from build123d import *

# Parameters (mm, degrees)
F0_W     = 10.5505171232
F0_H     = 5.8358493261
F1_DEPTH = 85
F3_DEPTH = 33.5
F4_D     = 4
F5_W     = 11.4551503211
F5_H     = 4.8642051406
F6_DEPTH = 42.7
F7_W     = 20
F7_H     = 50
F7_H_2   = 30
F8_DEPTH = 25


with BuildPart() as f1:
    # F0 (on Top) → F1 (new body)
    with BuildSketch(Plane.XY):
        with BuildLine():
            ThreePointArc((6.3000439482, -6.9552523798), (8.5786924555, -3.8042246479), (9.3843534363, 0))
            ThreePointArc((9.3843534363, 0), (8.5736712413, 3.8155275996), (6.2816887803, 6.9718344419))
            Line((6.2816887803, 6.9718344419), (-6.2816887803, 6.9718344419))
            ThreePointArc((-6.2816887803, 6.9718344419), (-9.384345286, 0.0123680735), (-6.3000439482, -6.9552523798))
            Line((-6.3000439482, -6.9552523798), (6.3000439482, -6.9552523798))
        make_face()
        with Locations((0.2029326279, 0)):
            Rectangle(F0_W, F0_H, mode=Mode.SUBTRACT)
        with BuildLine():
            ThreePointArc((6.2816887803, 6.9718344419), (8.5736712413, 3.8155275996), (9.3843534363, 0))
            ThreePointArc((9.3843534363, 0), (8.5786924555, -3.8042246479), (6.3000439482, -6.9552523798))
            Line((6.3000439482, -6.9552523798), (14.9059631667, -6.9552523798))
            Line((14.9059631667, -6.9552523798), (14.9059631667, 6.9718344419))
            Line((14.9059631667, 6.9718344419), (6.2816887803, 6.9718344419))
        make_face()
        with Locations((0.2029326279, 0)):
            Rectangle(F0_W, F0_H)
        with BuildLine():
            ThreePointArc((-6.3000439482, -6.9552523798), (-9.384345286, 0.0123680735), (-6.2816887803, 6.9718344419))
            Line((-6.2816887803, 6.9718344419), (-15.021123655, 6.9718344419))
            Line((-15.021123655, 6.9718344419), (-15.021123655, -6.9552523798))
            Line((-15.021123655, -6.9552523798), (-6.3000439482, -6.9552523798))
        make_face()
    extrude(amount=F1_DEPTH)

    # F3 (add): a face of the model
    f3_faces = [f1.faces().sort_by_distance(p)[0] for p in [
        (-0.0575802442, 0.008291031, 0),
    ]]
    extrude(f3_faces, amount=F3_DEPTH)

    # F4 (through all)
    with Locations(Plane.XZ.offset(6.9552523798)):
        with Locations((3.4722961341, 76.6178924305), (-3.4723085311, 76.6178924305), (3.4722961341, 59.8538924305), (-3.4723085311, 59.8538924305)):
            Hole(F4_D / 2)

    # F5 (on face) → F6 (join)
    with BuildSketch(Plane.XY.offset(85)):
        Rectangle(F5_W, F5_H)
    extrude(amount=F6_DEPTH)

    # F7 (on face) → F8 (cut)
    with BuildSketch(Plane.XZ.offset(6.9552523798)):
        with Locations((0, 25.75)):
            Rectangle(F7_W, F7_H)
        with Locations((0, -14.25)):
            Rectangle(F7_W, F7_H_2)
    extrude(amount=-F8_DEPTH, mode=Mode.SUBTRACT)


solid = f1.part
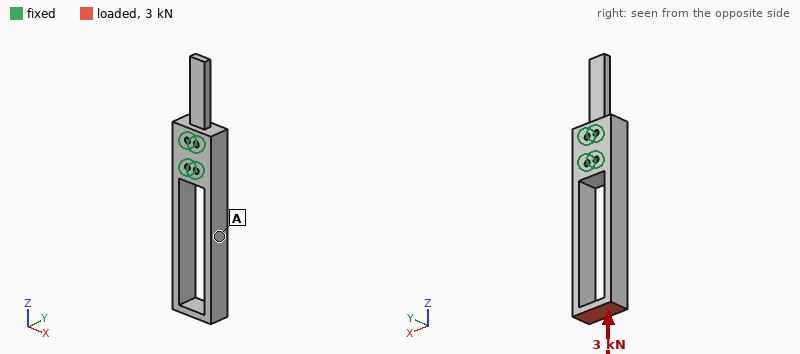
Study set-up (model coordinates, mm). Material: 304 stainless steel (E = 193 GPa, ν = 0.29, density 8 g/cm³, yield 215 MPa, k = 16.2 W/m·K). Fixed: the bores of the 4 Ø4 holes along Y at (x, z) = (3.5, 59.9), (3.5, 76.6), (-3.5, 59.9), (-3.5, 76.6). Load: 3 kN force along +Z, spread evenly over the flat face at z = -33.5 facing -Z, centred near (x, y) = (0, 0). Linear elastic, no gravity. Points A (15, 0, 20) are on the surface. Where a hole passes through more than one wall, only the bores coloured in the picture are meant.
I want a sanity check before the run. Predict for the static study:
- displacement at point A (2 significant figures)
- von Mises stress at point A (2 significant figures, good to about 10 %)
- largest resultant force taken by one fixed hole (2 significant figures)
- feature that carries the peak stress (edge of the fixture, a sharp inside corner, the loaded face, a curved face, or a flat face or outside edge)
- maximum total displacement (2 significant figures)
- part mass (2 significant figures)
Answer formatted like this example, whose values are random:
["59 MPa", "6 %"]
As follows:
["21 µm", "16 MPa", "920 N", "a flat face or outside edge", "30 µm", "230 g"]
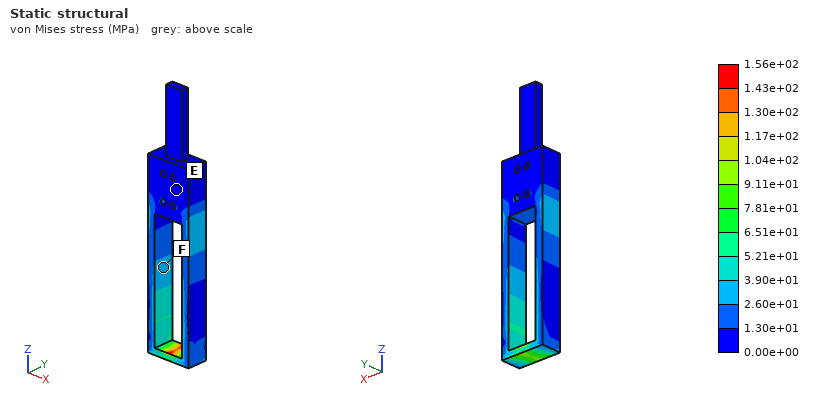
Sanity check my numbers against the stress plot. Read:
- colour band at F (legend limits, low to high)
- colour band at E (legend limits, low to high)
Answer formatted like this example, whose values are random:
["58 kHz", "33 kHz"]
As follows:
["2.60e+01 to 3.90e+01 MPa", "0.00e+00 to 1.30e+01 MPa"]
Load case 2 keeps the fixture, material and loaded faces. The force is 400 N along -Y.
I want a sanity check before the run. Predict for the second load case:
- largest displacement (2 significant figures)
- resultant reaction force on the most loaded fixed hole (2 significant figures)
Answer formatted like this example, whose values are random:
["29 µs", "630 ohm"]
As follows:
["0.25 mm", "580 N"]
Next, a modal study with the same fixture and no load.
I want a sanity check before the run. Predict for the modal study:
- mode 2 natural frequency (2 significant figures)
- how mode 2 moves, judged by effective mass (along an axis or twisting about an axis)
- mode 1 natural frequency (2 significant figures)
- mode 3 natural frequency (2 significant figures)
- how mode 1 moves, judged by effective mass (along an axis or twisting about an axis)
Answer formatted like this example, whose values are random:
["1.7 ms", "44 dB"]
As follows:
["1100 Hz", "along Y", "720 Hz", "2000 Hz", "along X"]
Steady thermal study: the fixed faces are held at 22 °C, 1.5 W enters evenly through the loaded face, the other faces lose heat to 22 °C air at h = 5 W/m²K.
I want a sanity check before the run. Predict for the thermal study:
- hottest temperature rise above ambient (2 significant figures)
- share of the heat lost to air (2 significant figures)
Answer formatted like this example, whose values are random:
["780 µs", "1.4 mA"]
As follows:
["42 K", "46 %"]
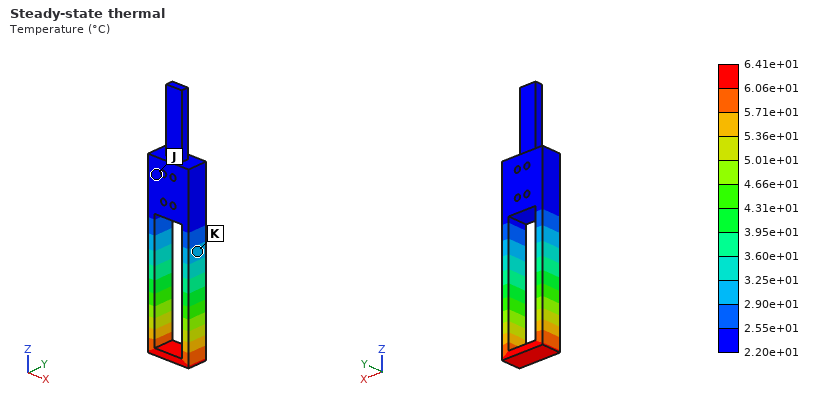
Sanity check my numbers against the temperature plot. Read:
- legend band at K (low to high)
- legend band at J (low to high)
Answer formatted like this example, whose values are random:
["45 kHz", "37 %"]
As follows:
["2.90e+01 to 3.25e+01 °C", "2.20e+01 to 2.55e+01 °C"]
